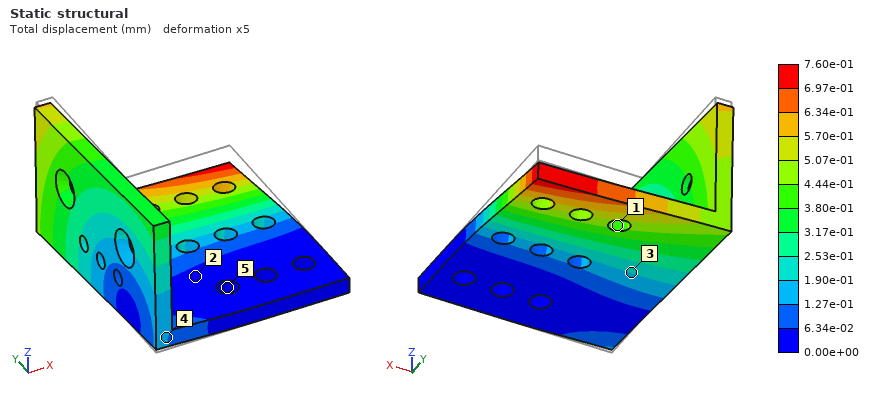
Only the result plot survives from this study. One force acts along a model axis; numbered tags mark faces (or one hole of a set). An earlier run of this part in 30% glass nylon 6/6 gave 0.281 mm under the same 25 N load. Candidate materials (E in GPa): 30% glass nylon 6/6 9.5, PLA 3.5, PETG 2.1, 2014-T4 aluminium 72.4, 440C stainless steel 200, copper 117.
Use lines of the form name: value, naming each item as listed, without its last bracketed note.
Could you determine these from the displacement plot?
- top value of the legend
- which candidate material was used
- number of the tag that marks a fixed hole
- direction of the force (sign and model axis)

top value of the legend: 7.60e-01 mm
which candidate material was used: PLA
number of the tag that marks a fixed hole: 5
direction of the force: -Z
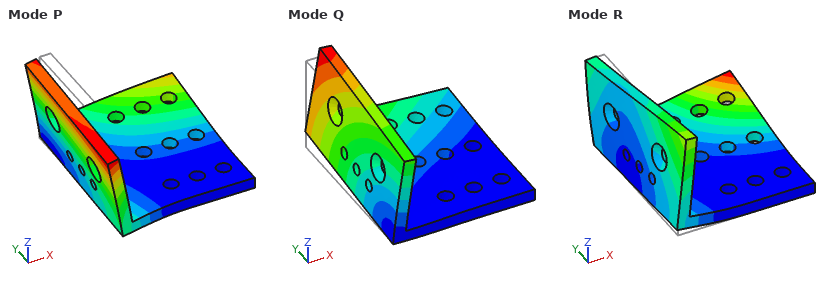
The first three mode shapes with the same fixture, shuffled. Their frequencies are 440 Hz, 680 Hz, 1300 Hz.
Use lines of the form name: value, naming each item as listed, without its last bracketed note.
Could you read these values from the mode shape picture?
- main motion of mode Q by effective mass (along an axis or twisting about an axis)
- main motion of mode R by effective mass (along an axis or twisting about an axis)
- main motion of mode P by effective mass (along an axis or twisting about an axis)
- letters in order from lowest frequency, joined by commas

main motion of mode Q by effective mass: along Z
main motion of mode R by effective mass: along Z
main motion of mode P by effective mass: along X
letters in order from lowest frequency, joined by commas: Q, P, R
